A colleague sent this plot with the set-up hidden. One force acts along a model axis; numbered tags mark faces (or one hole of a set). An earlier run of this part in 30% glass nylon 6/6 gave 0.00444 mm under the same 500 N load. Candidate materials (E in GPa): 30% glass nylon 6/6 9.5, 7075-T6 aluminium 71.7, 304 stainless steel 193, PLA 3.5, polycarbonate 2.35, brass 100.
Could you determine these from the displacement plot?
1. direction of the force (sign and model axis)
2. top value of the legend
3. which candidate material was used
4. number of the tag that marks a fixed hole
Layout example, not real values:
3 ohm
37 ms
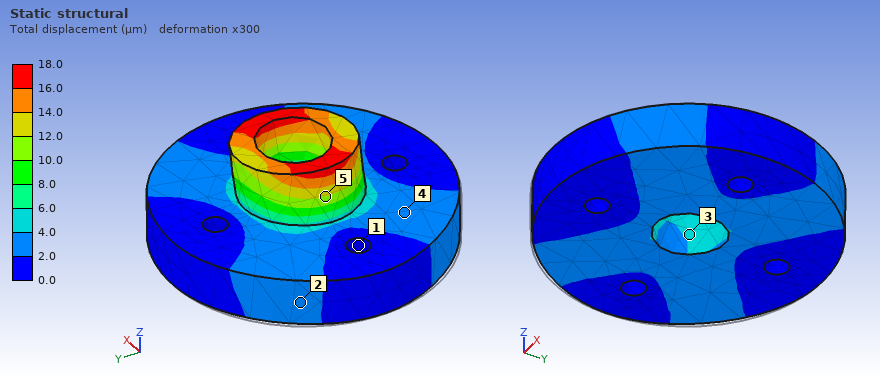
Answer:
+X
18.0 µm
polycarbonate
1
